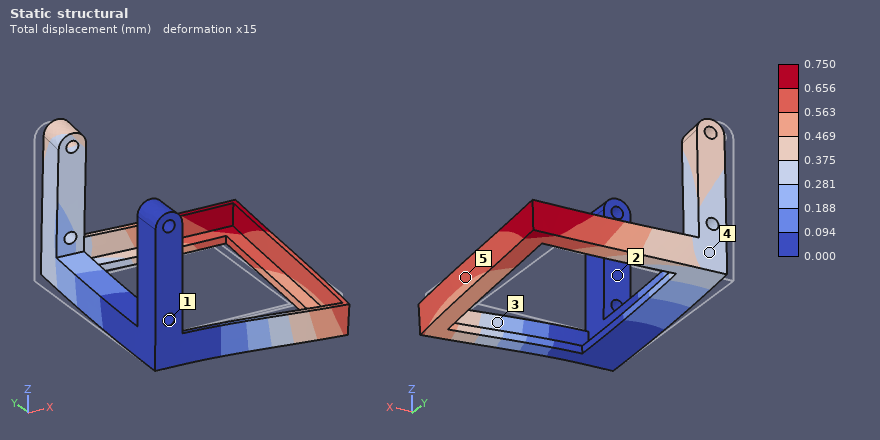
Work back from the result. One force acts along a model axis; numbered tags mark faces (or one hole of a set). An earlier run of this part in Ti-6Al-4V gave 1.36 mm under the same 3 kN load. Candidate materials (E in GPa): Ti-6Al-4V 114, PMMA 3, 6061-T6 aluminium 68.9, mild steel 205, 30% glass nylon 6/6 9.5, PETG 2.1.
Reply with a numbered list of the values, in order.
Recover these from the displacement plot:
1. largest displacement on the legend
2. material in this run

1. 0.750 mm
2. mild steel
